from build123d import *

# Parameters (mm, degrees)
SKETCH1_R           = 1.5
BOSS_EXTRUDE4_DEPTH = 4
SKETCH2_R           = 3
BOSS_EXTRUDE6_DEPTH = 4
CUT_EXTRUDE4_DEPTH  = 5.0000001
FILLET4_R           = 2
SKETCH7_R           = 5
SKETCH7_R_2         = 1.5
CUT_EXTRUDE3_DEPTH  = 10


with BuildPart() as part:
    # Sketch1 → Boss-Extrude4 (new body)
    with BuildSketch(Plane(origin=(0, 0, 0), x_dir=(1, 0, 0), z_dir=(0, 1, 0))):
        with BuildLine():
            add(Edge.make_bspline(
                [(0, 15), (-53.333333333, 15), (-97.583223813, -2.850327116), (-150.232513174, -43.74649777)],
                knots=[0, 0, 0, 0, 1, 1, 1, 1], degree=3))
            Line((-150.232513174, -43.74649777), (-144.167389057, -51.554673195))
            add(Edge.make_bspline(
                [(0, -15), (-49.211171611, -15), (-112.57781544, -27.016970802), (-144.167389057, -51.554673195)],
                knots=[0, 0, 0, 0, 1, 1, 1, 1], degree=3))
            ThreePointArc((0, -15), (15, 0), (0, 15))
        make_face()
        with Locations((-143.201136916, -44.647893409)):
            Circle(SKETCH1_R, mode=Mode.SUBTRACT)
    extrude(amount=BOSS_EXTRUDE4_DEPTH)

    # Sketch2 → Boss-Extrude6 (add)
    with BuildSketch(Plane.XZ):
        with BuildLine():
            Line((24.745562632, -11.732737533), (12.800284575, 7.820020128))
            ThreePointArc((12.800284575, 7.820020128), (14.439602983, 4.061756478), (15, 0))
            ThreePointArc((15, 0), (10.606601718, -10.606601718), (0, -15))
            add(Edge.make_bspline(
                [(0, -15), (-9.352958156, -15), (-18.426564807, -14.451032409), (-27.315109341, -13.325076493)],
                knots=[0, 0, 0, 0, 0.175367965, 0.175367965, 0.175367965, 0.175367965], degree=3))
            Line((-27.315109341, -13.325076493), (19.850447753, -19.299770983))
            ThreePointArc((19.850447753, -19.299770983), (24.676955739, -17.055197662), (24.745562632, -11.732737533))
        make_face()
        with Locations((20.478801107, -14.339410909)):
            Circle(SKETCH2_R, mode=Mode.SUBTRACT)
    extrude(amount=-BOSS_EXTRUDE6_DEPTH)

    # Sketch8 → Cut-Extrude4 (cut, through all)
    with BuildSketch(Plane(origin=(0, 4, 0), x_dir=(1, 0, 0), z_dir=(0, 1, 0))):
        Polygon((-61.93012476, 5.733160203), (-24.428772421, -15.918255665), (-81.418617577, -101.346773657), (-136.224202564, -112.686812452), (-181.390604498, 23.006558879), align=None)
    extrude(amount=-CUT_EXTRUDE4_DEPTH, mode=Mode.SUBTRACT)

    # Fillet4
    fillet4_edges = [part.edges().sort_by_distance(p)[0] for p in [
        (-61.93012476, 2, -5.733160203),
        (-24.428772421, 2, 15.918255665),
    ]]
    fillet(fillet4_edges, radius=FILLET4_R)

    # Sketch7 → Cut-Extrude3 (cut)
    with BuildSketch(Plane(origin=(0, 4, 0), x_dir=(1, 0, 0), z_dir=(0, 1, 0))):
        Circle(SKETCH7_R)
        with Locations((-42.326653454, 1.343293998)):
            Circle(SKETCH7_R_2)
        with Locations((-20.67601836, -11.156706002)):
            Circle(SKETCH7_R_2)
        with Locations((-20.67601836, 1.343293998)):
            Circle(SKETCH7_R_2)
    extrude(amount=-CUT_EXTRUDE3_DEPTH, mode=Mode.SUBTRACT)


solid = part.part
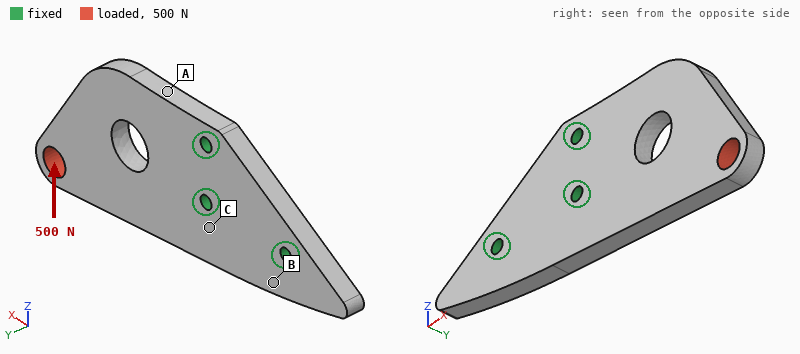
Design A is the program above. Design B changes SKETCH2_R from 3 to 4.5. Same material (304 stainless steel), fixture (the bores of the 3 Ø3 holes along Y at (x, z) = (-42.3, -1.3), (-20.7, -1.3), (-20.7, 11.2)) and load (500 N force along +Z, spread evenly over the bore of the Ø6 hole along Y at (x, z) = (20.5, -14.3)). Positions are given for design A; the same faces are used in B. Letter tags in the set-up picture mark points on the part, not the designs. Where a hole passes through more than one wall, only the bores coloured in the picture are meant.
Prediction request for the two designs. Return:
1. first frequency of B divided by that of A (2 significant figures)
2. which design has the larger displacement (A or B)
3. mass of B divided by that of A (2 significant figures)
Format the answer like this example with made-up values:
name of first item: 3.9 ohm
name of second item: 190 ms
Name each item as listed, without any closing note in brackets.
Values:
first frequency of B divided by that of A: 1.1
which design has the larger displacement: B
mass of B divided by that of A: 0.98
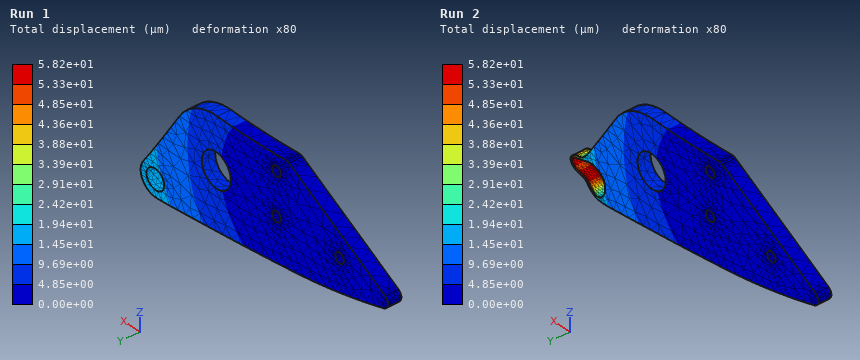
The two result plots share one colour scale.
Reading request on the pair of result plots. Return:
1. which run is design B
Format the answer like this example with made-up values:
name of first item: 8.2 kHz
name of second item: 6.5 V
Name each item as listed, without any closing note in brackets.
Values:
which run is design B: Run 2
